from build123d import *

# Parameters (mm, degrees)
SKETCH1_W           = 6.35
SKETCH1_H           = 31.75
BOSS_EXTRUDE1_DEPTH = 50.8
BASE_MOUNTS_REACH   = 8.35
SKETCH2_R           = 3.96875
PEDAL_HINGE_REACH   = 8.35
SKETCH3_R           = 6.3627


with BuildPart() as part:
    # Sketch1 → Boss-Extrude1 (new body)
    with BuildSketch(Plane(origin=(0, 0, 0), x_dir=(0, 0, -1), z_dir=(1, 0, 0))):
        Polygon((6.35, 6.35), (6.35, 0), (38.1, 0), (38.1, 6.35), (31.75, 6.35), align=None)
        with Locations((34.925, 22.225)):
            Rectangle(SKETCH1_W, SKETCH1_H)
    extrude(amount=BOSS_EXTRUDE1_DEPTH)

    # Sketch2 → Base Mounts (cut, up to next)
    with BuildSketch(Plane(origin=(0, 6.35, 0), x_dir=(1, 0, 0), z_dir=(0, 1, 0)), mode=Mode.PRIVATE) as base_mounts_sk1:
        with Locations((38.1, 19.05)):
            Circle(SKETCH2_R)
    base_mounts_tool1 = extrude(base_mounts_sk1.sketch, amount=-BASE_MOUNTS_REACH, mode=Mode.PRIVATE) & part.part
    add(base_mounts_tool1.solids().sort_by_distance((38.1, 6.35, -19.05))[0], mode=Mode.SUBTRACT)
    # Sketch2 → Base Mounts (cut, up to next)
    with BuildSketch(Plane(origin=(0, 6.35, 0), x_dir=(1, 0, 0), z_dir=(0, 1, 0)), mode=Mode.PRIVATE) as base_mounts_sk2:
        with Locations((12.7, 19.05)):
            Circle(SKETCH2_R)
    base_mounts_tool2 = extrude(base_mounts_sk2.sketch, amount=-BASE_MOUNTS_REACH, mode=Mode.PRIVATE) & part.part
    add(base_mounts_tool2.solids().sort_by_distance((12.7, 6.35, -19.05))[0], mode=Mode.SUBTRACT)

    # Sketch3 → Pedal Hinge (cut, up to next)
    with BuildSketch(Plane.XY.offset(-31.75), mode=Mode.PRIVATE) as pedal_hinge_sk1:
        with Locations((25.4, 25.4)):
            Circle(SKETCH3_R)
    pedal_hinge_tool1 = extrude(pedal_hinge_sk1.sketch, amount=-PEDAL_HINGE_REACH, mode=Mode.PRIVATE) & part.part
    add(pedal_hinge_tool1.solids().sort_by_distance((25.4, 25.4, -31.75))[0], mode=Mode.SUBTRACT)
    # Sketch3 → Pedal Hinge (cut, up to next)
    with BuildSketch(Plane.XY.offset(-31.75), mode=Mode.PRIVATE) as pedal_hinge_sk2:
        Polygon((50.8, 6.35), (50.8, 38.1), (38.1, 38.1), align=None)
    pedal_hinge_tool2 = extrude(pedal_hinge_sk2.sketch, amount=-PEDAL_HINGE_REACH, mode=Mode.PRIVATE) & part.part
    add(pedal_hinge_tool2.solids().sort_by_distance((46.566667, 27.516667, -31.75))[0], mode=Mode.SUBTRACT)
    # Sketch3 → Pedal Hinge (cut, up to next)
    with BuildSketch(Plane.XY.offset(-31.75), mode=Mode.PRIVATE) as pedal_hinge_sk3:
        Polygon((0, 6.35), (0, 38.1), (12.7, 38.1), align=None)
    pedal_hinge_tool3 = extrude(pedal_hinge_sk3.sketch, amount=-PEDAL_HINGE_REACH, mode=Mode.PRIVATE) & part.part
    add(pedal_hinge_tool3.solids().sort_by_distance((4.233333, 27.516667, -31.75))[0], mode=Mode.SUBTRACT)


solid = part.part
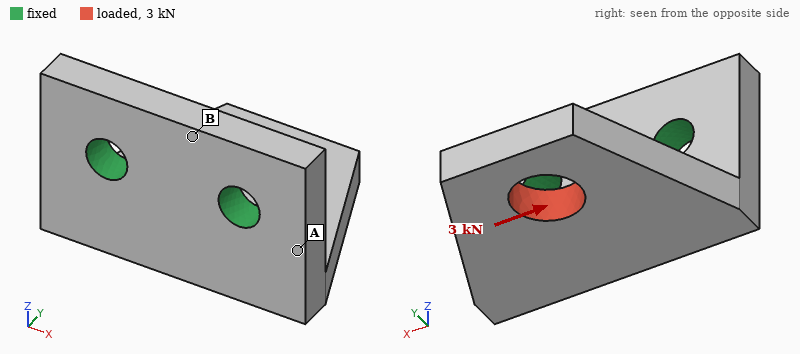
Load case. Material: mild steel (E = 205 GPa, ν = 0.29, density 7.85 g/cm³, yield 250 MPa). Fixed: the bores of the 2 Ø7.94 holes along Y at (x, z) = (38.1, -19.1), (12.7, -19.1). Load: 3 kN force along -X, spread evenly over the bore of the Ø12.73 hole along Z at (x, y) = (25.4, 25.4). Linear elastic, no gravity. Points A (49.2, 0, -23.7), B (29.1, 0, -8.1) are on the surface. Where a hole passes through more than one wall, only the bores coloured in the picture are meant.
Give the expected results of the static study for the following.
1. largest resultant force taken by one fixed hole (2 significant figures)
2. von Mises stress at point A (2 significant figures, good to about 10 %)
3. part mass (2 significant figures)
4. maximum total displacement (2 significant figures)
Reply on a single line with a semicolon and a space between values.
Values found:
2.9 kN; 61 MPa; 130 g; 40 µm
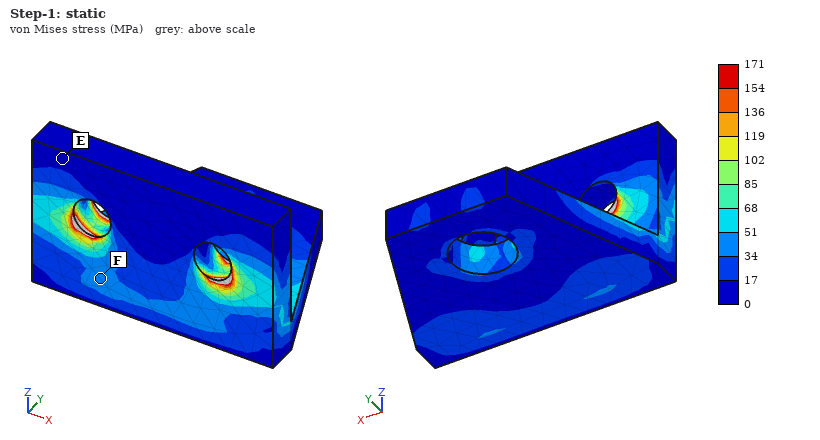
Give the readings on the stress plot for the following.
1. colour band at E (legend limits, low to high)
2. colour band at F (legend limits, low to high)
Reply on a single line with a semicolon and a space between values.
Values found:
0 to 17 MPa; 34 to 51 MPa
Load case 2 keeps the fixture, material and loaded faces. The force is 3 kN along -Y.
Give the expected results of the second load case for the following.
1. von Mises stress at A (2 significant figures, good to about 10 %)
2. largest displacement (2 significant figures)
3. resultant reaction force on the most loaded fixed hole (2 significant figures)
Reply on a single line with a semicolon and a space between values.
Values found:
57 MPa; 53 µm; 1.5 kN
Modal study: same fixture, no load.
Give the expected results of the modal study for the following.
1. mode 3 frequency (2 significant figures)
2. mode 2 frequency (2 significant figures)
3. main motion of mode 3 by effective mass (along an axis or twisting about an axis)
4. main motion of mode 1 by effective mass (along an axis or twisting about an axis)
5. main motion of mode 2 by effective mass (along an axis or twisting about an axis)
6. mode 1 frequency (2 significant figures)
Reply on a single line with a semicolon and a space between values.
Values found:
11 kHz; 7200 Hz; along Y; along Z; along X; 3500 Hz
